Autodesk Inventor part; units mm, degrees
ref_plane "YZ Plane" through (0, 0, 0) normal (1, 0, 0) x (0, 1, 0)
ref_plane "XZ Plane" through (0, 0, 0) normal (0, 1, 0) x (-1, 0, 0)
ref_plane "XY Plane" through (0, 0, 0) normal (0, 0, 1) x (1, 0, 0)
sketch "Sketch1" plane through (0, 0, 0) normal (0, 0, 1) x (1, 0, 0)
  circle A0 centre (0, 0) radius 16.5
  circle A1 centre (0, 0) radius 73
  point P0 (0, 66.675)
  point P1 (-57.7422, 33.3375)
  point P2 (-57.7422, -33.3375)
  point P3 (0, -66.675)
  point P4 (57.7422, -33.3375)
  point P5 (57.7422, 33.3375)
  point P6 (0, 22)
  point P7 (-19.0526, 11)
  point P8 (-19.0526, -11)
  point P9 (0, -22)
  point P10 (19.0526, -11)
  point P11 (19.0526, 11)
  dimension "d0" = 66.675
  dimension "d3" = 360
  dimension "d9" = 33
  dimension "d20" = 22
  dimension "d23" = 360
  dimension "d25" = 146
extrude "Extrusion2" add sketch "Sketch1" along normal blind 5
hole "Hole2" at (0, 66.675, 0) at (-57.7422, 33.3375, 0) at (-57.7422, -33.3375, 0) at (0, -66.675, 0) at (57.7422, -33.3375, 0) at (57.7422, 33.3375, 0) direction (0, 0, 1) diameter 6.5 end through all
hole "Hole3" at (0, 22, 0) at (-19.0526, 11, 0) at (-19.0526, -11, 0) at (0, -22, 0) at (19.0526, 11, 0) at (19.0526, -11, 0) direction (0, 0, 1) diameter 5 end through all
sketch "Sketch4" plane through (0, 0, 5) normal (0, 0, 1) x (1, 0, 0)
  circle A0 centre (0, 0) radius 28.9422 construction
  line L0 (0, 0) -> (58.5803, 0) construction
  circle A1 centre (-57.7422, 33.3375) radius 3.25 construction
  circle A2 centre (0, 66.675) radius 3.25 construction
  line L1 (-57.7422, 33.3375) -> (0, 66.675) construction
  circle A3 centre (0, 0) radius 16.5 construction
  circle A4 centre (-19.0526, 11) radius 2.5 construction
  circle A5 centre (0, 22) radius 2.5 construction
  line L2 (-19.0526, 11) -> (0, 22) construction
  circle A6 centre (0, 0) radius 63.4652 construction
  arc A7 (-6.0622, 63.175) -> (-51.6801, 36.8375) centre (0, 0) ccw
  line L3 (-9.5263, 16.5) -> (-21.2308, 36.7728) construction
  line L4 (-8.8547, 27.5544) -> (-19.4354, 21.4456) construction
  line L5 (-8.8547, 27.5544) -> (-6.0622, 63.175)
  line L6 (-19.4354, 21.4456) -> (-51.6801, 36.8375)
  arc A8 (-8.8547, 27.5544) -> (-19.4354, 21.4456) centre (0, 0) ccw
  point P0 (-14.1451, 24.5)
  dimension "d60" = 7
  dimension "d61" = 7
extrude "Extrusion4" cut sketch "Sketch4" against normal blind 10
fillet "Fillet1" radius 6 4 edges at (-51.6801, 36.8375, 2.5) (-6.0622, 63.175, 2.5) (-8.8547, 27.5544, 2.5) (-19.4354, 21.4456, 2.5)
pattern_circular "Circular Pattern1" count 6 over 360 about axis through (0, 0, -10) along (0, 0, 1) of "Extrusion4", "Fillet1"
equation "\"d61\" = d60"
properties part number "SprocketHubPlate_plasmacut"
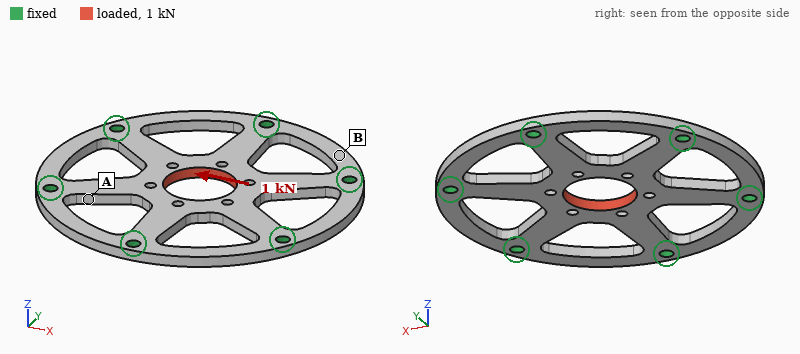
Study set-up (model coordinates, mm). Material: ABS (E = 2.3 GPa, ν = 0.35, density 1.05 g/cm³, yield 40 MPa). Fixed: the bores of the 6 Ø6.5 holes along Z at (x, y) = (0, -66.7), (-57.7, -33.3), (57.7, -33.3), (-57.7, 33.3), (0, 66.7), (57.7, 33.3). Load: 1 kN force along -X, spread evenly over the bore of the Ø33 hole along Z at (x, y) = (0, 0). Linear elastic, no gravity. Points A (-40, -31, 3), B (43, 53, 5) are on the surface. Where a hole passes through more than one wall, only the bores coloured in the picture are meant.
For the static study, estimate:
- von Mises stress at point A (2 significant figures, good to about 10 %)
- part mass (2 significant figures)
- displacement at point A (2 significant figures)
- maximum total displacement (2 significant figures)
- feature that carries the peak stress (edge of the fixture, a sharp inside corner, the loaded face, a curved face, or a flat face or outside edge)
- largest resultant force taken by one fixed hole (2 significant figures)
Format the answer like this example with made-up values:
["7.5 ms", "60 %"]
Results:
["3.5 MPa", "46 g", "21 µm", "88 µm", "a curved face", "260 N"]
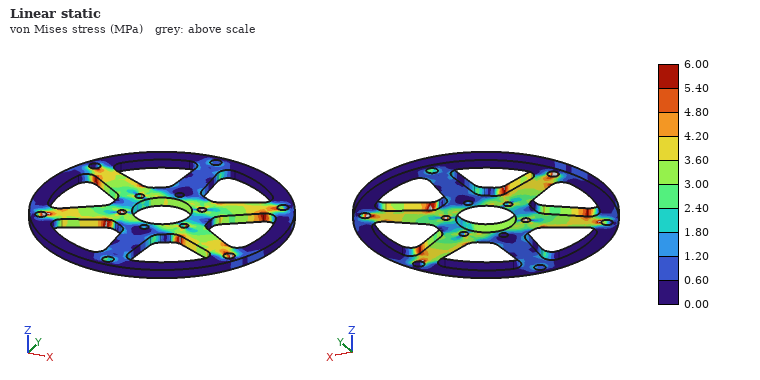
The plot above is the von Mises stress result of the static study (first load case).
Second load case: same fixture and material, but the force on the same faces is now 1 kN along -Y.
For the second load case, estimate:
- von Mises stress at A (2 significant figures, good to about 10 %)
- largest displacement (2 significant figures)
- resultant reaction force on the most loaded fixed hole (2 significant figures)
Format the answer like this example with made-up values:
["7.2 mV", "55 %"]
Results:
["2.7 MPa", "87 µm", "300 N"]
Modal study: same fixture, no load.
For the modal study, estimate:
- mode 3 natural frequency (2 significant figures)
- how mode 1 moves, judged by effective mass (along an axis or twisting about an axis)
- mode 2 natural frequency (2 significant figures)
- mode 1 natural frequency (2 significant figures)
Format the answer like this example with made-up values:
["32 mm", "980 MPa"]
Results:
["1200 Hz", "along Z", "1200 Hz", "600 Hz"]
